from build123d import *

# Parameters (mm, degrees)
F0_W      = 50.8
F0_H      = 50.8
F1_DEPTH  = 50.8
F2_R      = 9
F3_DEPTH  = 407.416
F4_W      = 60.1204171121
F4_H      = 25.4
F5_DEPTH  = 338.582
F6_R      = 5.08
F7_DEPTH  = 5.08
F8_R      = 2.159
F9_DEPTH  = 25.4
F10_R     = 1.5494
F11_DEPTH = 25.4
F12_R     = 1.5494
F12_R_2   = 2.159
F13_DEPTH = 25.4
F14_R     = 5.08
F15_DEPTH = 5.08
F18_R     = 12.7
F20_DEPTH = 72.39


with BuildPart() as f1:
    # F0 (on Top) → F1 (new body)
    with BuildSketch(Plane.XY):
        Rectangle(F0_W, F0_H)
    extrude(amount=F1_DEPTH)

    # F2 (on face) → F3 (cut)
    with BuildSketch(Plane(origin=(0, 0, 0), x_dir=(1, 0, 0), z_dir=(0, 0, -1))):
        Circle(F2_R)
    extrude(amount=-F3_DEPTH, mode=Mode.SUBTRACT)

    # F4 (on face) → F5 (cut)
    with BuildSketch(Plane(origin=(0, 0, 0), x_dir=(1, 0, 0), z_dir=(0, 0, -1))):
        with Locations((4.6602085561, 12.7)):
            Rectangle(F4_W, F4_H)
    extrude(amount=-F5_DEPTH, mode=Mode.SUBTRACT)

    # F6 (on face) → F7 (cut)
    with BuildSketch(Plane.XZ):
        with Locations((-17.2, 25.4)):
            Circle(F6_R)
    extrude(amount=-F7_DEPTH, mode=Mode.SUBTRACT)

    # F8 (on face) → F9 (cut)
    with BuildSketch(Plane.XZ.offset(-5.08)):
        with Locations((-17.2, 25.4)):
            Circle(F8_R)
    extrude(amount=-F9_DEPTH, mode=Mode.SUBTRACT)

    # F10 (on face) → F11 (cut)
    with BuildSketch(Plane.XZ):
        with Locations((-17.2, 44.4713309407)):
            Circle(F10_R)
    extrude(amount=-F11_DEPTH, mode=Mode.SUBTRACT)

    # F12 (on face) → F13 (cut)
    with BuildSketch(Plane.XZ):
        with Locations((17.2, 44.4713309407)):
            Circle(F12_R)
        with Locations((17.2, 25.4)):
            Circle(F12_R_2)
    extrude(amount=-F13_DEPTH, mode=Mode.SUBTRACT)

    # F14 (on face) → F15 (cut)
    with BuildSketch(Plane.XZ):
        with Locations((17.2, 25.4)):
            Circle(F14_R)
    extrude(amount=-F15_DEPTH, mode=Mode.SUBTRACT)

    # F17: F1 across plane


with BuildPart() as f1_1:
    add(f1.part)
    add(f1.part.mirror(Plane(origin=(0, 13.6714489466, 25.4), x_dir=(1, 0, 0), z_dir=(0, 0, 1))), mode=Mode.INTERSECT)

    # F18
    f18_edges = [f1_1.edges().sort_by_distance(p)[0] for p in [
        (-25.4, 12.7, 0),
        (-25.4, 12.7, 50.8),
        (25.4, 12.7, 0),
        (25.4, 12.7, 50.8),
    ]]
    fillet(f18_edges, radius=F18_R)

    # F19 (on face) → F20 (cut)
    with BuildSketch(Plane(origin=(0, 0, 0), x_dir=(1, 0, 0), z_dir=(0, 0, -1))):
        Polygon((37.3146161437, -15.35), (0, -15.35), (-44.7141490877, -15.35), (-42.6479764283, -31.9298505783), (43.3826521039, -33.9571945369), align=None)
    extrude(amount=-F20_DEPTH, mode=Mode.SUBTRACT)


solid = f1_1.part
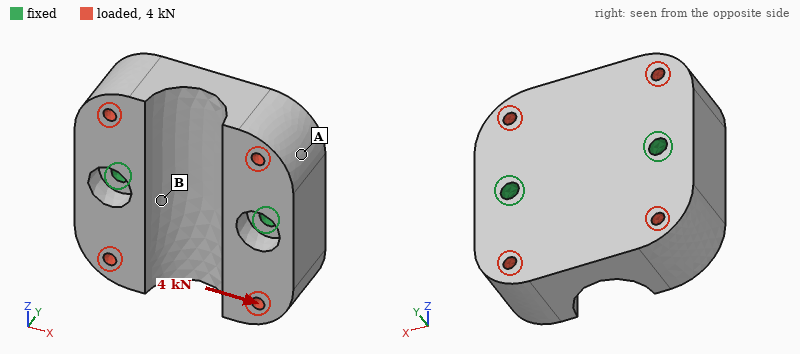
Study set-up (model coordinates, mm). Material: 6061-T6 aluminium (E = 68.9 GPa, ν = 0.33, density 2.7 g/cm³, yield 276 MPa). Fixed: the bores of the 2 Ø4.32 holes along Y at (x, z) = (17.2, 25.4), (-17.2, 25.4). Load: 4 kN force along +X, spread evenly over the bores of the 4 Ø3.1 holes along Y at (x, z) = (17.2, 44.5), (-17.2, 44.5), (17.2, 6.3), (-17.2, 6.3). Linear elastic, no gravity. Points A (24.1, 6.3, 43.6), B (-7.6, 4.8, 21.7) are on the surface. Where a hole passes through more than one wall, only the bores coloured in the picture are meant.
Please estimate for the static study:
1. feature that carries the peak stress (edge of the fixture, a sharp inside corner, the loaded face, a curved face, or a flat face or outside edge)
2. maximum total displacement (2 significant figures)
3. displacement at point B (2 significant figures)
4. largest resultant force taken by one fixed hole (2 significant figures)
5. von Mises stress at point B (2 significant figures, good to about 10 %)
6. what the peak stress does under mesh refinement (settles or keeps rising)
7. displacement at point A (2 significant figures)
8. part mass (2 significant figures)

edge of the fixture
6.3 µm
1.6 µm
2.0 kN
8.6 MPa
keeps rising
5.0 µm
79 g
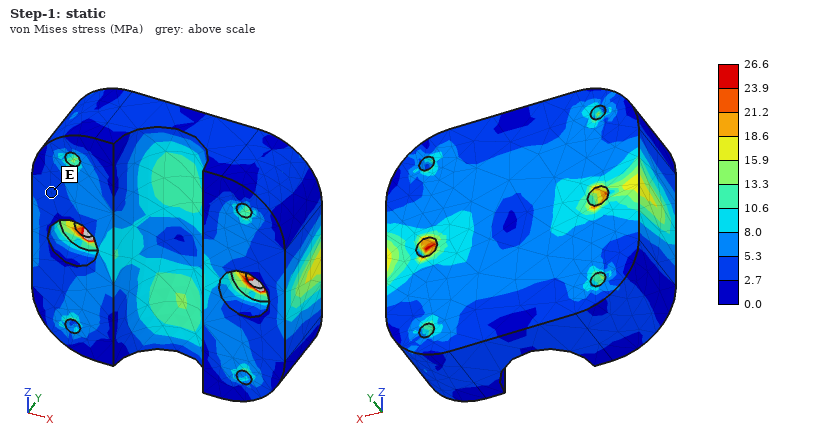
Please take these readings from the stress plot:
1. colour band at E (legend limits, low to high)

2.7 to 5.3 MPa
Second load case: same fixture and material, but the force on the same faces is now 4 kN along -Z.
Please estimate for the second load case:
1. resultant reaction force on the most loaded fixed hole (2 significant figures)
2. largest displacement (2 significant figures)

2.0 kN
6.1 µm
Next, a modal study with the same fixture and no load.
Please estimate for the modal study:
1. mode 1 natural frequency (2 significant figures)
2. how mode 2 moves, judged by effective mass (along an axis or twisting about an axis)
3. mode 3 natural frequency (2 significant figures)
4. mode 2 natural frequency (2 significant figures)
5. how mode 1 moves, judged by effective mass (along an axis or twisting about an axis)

8800 Hz
along Y
15 kHz
14 kHz
twisting about X
